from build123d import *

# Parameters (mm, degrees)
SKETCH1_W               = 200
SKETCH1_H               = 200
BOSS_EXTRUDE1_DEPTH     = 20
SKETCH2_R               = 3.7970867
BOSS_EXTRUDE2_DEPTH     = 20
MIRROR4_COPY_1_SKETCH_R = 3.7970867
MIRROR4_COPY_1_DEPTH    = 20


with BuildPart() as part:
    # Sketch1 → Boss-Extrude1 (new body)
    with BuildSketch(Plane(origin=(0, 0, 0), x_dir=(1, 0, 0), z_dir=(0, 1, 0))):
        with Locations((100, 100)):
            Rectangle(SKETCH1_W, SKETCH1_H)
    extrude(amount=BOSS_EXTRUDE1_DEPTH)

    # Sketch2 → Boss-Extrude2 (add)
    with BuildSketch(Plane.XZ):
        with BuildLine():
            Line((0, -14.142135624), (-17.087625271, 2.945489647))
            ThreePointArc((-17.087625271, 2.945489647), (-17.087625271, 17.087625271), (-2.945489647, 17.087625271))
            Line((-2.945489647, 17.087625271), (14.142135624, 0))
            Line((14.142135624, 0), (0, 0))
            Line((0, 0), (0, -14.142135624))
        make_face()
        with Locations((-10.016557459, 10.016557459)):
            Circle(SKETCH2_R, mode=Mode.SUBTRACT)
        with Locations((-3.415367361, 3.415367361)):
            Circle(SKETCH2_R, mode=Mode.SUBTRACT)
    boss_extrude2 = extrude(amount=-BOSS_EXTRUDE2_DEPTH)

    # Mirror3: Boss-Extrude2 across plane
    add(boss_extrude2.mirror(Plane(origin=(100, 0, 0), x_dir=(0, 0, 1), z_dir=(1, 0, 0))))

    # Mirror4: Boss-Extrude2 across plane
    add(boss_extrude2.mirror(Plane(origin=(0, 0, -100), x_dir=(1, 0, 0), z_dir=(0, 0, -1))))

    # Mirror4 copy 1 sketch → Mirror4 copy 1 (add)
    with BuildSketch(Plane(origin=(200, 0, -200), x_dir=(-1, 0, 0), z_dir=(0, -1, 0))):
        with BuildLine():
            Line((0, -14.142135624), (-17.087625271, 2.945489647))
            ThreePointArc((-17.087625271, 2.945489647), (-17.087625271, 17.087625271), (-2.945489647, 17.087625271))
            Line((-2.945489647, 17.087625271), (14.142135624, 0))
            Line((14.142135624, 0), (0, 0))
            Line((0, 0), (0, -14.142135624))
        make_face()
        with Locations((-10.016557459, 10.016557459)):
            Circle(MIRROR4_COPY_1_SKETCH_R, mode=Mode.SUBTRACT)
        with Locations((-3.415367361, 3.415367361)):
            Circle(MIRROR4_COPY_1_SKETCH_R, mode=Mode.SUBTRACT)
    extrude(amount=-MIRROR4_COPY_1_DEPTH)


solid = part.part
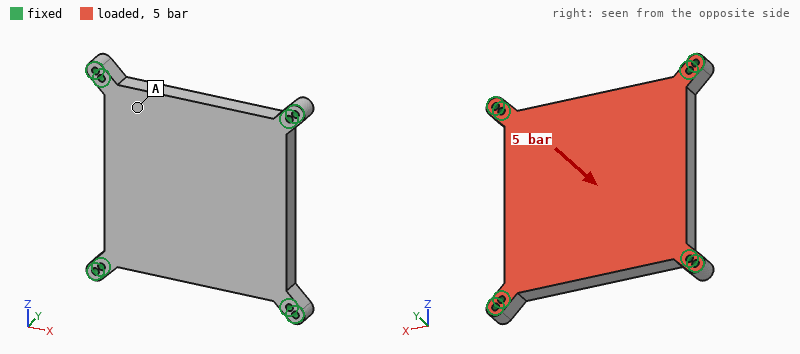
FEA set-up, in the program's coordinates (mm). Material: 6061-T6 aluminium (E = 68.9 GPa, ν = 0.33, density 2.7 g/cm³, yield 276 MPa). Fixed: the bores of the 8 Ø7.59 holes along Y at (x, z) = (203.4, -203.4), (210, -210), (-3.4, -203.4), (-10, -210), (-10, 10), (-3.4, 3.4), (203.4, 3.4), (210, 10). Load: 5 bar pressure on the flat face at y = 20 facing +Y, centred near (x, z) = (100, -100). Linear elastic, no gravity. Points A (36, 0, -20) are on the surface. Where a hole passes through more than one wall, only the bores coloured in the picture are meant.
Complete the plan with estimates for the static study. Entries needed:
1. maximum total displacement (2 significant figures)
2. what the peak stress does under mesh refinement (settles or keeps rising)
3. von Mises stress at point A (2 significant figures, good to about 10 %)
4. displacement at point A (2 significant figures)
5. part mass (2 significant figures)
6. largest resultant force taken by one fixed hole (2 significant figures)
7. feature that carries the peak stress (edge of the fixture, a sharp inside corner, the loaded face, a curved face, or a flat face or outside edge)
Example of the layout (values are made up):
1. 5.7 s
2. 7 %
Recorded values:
1. 0.21 mm
2. keeps rising
3. 13 MPa
4. 0.096 mm
5. 2.3 kg
6. 6.0 kN
7. edge of the fixture
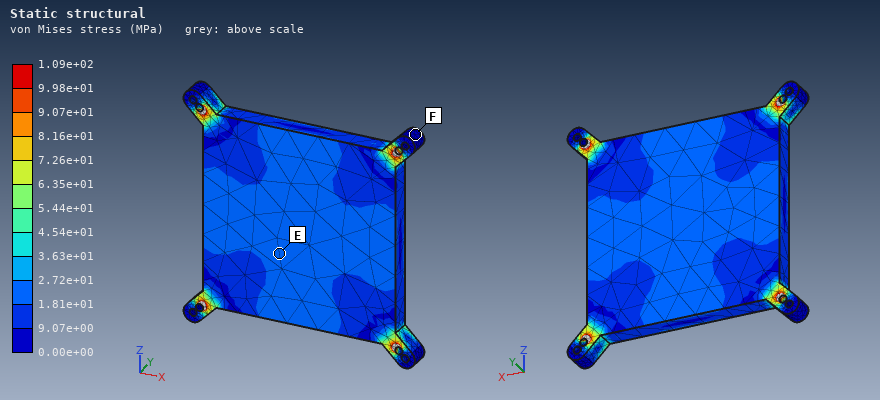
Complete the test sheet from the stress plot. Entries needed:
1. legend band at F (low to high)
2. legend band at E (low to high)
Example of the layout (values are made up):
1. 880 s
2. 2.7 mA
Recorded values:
1. 0.00e+00 to 9.07e+00 MPa
2. 1.81e+01 to 2.72e+01 MPa
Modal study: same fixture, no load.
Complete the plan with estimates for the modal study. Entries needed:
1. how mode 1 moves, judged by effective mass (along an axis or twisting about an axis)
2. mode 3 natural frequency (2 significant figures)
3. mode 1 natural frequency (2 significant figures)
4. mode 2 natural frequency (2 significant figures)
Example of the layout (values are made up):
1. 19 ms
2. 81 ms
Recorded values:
1. along Y
2. 2200 Hz
3. 1200 Hz
4. 2200 Hz
